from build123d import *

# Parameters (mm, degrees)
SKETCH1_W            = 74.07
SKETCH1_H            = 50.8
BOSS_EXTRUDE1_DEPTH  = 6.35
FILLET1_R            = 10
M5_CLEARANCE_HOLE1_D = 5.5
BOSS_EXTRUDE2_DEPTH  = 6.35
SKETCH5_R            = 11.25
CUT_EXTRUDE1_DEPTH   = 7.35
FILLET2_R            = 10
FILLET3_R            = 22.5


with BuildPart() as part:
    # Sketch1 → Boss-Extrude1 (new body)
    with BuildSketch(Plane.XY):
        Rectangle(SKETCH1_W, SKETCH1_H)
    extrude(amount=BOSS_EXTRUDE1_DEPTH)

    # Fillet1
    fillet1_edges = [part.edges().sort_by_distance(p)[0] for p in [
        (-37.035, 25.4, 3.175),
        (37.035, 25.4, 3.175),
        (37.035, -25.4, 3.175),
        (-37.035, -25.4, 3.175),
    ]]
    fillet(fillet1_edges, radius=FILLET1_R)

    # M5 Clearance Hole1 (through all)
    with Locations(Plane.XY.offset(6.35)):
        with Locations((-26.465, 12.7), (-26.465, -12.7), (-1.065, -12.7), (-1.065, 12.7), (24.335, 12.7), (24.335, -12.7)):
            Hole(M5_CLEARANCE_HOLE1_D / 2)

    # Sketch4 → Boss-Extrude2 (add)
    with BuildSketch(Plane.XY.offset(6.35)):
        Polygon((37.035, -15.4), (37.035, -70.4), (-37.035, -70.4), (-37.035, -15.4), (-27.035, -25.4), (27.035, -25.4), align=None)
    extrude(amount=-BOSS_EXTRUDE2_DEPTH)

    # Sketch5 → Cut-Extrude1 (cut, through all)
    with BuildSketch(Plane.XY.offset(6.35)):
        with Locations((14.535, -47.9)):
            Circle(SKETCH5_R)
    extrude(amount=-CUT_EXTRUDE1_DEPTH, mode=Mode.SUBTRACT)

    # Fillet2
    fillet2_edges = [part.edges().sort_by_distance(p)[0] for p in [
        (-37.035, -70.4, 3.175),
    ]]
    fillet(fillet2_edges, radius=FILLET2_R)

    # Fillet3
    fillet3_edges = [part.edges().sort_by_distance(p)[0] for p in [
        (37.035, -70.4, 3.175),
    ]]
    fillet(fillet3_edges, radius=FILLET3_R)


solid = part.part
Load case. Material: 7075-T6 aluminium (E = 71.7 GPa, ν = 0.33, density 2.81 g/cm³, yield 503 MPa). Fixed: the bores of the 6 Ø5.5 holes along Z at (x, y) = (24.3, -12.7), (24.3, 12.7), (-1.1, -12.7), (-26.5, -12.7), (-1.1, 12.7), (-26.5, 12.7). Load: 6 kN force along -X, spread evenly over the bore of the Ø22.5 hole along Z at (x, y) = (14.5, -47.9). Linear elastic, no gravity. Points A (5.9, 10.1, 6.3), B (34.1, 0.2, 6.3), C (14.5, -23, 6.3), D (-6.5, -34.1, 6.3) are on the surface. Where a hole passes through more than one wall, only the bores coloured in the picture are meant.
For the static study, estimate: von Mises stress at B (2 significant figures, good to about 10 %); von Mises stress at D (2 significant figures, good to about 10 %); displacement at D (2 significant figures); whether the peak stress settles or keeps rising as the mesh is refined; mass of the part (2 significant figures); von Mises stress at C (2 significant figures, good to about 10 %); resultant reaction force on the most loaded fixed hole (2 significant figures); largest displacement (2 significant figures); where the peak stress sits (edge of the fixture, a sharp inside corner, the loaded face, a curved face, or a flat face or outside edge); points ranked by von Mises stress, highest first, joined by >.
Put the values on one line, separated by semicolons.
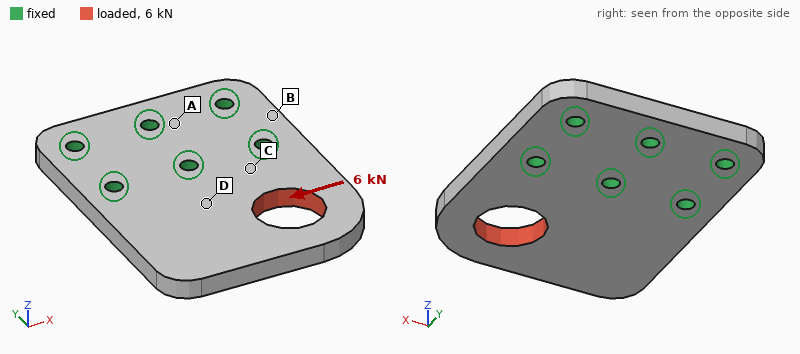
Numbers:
12 MPa; 23 MPa; 14 µm; keeps rising; 110 g; 41 MPa; 3.7 kN; 51 µm; edge of the fixture; C > D > B > A
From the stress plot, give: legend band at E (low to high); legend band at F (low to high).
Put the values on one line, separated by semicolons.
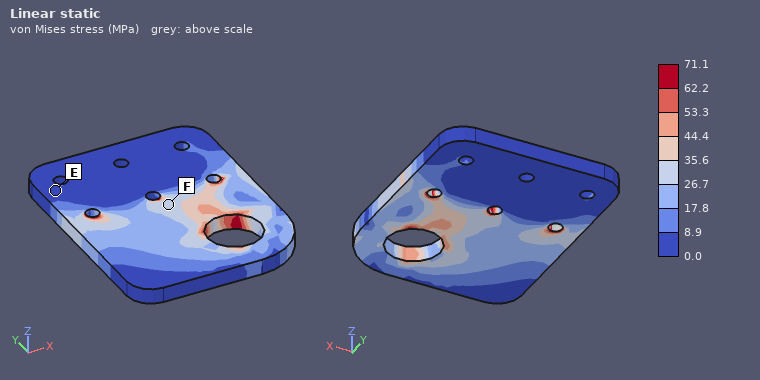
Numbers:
0.0 to 8.9 MPa; 26.7 to 35.6 MPa
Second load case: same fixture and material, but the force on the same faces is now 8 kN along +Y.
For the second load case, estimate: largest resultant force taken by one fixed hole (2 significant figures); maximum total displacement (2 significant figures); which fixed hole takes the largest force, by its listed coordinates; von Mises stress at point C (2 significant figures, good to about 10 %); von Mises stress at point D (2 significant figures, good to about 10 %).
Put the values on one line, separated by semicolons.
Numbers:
4.2 kN; 33 µm; (24.3, -12.7); 20 MPa; 20 MPa
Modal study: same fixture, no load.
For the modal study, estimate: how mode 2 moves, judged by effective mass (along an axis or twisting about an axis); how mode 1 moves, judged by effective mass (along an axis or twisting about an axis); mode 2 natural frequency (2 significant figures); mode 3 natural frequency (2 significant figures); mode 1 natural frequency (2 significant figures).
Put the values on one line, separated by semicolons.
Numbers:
twisting about Y; along Z; 3400 Hz; 7400 Hz; 1700 Hz
